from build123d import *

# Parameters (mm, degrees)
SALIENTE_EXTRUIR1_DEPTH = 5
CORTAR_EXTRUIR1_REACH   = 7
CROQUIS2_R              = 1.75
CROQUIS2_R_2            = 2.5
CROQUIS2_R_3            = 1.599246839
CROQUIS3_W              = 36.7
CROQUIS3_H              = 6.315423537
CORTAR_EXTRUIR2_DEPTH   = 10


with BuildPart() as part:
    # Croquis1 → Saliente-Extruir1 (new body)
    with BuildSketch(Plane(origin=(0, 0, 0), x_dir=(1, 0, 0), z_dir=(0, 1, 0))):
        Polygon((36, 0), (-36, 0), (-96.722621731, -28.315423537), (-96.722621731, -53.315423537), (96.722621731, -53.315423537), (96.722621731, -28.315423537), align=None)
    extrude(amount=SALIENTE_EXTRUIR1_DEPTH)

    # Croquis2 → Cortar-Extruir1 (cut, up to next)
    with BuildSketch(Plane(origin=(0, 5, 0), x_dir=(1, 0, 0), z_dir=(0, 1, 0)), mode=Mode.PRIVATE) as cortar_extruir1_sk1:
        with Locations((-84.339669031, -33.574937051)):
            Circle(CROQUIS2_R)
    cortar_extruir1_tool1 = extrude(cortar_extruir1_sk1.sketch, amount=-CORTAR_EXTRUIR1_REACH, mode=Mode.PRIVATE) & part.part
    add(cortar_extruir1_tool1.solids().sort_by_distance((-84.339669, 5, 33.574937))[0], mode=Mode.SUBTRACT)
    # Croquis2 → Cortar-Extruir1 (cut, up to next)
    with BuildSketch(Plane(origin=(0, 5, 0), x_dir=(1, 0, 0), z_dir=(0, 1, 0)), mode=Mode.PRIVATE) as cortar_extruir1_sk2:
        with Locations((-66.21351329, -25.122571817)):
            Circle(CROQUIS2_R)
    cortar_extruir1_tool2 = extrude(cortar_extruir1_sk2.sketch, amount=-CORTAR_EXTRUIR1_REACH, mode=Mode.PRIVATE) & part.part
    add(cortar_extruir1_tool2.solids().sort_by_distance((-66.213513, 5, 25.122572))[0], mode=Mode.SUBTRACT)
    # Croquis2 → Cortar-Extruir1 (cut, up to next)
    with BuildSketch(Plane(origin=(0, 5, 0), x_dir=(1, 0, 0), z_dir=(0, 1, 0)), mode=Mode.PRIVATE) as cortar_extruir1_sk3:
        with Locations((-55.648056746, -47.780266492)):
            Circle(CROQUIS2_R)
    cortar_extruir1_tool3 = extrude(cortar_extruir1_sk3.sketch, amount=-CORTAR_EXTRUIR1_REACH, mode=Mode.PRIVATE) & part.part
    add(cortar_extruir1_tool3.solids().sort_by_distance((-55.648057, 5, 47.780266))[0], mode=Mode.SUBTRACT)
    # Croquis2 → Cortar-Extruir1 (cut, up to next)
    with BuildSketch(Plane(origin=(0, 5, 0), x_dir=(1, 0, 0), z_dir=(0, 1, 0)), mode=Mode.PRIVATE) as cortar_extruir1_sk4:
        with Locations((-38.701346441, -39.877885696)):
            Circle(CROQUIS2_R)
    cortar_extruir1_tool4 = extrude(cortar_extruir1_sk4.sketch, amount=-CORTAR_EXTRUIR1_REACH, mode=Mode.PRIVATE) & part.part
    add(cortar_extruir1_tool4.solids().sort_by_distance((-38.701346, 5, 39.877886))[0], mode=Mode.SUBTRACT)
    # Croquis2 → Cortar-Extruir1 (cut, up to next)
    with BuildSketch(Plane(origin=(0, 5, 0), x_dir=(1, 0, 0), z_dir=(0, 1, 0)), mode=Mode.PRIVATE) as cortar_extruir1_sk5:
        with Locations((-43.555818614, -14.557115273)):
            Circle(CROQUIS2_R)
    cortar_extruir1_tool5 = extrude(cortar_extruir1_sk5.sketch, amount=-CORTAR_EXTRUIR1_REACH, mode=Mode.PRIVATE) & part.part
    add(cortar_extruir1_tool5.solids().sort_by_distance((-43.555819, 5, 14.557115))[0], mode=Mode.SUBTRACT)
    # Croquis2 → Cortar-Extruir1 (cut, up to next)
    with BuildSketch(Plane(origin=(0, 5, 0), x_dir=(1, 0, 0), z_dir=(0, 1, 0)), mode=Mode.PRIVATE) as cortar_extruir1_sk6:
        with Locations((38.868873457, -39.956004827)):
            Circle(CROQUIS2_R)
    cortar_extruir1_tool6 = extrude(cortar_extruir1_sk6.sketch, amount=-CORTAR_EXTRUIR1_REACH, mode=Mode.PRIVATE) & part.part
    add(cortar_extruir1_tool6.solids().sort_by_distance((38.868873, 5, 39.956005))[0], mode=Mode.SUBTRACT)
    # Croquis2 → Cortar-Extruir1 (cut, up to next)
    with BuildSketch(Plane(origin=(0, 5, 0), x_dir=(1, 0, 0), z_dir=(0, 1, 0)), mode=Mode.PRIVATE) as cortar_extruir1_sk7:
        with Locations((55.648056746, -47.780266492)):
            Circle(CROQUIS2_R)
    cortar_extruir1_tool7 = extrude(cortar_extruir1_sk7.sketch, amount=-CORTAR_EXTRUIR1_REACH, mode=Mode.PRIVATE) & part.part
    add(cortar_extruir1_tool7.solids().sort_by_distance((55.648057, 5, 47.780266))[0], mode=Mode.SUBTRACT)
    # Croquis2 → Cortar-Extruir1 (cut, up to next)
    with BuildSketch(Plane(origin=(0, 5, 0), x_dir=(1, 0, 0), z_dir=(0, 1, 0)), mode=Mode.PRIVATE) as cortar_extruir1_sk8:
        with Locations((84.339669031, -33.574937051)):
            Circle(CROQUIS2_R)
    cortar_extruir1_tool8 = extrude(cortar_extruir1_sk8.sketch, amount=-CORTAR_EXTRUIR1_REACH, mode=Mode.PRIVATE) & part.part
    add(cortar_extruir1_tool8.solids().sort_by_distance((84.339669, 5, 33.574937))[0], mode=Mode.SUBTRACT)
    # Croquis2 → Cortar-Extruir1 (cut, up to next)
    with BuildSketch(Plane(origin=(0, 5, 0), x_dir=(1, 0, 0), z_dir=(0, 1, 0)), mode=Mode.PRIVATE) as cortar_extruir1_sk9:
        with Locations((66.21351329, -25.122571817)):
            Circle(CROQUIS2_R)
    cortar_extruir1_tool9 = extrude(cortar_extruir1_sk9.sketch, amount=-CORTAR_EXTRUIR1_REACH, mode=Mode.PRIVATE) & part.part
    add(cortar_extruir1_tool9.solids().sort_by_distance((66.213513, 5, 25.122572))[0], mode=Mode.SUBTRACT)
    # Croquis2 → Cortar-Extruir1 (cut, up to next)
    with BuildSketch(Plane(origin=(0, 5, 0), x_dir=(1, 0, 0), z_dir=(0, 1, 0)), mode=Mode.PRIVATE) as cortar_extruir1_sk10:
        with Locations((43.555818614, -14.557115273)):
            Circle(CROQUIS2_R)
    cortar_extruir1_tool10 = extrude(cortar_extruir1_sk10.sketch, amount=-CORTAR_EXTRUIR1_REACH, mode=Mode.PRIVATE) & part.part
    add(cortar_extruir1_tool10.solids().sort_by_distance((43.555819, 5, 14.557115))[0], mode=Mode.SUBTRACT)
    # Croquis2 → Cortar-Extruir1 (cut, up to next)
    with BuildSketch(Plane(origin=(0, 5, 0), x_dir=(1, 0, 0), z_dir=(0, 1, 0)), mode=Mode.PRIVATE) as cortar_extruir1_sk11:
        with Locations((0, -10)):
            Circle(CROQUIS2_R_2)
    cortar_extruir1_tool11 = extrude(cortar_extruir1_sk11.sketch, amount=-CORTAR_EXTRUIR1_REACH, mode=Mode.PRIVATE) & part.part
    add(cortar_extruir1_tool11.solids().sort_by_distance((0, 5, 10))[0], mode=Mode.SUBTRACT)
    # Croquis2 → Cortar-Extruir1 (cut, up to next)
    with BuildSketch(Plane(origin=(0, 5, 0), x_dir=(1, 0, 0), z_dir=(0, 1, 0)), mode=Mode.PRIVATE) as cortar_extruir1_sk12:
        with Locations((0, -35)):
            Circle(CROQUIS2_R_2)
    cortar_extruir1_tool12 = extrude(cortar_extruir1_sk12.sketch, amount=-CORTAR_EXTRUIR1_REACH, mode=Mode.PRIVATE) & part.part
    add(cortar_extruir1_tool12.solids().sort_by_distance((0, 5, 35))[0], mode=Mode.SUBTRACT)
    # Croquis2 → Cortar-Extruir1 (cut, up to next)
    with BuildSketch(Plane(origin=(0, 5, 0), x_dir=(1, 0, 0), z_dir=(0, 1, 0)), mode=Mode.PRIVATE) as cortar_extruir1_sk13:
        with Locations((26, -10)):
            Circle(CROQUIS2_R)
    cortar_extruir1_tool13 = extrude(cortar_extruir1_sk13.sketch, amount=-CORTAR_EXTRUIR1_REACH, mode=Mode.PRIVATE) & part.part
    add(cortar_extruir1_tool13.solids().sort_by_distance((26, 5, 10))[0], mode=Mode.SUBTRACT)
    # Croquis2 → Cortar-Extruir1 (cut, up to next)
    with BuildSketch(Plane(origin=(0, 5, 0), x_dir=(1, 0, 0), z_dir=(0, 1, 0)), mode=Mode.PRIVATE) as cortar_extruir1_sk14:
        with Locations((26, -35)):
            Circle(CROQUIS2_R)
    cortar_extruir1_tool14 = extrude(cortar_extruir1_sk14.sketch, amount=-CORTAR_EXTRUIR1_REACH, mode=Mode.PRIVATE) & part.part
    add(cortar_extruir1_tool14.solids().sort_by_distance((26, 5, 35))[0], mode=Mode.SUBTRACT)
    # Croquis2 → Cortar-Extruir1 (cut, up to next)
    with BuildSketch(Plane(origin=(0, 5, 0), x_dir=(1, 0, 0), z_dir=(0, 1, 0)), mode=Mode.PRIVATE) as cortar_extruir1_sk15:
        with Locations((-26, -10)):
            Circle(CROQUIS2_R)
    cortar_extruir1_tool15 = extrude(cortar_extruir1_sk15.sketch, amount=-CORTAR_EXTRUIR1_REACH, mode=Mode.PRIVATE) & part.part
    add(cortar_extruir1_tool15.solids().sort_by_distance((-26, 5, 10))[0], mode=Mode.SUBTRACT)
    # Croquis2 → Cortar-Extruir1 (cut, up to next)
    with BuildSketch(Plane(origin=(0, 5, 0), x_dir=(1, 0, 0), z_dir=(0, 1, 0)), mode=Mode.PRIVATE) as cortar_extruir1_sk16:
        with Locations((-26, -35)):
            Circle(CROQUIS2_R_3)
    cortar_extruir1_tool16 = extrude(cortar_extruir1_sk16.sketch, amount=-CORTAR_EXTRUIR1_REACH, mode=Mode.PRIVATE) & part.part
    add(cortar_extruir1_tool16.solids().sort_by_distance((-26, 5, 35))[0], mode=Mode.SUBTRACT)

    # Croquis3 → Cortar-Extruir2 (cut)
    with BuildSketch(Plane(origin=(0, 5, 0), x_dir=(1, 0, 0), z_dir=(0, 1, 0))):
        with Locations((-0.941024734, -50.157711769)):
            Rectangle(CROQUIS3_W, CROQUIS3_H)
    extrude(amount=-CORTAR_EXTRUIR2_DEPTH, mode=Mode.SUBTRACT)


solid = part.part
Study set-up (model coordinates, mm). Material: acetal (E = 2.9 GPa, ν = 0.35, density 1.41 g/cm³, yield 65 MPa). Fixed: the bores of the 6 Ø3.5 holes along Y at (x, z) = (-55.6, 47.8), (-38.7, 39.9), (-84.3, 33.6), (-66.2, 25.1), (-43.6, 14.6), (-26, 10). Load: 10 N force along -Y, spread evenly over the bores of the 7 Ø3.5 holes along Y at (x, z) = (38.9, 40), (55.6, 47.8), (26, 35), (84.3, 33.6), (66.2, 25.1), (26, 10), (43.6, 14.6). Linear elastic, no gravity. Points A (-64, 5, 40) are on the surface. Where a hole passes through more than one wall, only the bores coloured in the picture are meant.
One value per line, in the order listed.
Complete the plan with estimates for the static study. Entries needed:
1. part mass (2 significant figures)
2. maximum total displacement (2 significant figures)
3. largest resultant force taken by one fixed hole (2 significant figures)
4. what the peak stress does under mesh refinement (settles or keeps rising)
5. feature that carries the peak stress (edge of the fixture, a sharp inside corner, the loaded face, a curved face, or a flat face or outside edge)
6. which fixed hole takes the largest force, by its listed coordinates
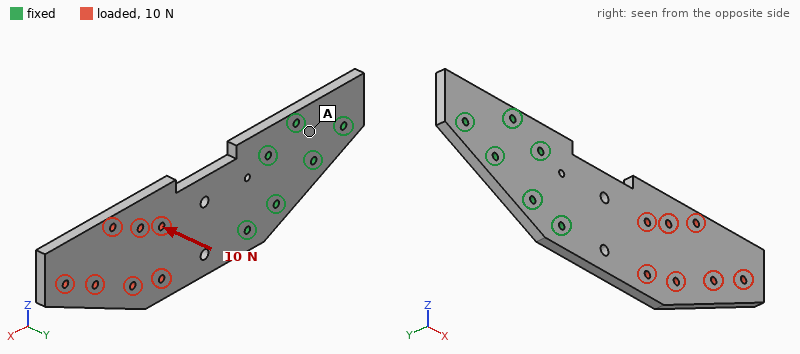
58 g
2.4 mm
22 N
keeps rising
edge of the fixture
(-26, 10)
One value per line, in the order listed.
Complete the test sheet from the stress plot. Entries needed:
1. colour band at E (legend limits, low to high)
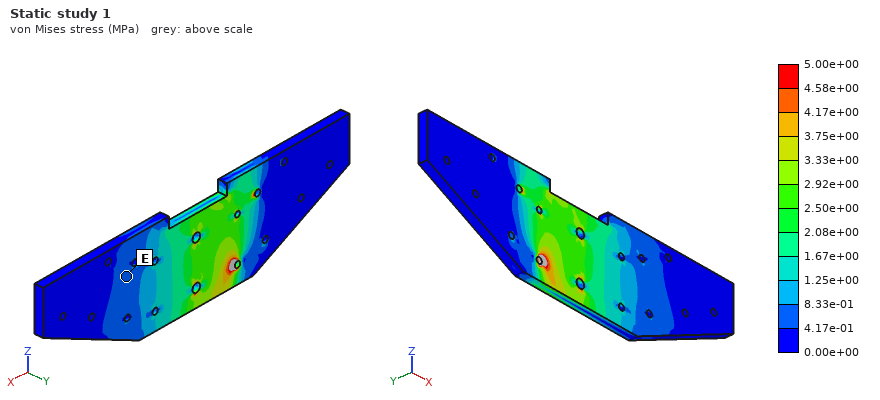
4.17e-01 to 8.33e-01 MPa
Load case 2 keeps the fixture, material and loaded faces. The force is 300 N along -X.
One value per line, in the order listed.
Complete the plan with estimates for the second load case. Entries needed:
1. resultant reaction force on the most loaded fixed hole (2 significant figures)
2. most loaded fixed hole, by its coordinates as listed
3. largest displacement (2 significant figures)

130 N
(-38.7, 39.9)
0.13 mm
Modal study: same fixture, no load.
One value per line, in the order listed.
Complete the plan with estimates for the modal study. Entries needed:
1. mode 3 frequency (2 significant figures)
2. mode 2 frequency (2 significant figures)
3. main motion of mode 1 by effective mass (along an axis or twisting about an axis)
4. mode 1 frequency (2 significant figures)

470 Hz
440 Hz
along Y
81 Hz
